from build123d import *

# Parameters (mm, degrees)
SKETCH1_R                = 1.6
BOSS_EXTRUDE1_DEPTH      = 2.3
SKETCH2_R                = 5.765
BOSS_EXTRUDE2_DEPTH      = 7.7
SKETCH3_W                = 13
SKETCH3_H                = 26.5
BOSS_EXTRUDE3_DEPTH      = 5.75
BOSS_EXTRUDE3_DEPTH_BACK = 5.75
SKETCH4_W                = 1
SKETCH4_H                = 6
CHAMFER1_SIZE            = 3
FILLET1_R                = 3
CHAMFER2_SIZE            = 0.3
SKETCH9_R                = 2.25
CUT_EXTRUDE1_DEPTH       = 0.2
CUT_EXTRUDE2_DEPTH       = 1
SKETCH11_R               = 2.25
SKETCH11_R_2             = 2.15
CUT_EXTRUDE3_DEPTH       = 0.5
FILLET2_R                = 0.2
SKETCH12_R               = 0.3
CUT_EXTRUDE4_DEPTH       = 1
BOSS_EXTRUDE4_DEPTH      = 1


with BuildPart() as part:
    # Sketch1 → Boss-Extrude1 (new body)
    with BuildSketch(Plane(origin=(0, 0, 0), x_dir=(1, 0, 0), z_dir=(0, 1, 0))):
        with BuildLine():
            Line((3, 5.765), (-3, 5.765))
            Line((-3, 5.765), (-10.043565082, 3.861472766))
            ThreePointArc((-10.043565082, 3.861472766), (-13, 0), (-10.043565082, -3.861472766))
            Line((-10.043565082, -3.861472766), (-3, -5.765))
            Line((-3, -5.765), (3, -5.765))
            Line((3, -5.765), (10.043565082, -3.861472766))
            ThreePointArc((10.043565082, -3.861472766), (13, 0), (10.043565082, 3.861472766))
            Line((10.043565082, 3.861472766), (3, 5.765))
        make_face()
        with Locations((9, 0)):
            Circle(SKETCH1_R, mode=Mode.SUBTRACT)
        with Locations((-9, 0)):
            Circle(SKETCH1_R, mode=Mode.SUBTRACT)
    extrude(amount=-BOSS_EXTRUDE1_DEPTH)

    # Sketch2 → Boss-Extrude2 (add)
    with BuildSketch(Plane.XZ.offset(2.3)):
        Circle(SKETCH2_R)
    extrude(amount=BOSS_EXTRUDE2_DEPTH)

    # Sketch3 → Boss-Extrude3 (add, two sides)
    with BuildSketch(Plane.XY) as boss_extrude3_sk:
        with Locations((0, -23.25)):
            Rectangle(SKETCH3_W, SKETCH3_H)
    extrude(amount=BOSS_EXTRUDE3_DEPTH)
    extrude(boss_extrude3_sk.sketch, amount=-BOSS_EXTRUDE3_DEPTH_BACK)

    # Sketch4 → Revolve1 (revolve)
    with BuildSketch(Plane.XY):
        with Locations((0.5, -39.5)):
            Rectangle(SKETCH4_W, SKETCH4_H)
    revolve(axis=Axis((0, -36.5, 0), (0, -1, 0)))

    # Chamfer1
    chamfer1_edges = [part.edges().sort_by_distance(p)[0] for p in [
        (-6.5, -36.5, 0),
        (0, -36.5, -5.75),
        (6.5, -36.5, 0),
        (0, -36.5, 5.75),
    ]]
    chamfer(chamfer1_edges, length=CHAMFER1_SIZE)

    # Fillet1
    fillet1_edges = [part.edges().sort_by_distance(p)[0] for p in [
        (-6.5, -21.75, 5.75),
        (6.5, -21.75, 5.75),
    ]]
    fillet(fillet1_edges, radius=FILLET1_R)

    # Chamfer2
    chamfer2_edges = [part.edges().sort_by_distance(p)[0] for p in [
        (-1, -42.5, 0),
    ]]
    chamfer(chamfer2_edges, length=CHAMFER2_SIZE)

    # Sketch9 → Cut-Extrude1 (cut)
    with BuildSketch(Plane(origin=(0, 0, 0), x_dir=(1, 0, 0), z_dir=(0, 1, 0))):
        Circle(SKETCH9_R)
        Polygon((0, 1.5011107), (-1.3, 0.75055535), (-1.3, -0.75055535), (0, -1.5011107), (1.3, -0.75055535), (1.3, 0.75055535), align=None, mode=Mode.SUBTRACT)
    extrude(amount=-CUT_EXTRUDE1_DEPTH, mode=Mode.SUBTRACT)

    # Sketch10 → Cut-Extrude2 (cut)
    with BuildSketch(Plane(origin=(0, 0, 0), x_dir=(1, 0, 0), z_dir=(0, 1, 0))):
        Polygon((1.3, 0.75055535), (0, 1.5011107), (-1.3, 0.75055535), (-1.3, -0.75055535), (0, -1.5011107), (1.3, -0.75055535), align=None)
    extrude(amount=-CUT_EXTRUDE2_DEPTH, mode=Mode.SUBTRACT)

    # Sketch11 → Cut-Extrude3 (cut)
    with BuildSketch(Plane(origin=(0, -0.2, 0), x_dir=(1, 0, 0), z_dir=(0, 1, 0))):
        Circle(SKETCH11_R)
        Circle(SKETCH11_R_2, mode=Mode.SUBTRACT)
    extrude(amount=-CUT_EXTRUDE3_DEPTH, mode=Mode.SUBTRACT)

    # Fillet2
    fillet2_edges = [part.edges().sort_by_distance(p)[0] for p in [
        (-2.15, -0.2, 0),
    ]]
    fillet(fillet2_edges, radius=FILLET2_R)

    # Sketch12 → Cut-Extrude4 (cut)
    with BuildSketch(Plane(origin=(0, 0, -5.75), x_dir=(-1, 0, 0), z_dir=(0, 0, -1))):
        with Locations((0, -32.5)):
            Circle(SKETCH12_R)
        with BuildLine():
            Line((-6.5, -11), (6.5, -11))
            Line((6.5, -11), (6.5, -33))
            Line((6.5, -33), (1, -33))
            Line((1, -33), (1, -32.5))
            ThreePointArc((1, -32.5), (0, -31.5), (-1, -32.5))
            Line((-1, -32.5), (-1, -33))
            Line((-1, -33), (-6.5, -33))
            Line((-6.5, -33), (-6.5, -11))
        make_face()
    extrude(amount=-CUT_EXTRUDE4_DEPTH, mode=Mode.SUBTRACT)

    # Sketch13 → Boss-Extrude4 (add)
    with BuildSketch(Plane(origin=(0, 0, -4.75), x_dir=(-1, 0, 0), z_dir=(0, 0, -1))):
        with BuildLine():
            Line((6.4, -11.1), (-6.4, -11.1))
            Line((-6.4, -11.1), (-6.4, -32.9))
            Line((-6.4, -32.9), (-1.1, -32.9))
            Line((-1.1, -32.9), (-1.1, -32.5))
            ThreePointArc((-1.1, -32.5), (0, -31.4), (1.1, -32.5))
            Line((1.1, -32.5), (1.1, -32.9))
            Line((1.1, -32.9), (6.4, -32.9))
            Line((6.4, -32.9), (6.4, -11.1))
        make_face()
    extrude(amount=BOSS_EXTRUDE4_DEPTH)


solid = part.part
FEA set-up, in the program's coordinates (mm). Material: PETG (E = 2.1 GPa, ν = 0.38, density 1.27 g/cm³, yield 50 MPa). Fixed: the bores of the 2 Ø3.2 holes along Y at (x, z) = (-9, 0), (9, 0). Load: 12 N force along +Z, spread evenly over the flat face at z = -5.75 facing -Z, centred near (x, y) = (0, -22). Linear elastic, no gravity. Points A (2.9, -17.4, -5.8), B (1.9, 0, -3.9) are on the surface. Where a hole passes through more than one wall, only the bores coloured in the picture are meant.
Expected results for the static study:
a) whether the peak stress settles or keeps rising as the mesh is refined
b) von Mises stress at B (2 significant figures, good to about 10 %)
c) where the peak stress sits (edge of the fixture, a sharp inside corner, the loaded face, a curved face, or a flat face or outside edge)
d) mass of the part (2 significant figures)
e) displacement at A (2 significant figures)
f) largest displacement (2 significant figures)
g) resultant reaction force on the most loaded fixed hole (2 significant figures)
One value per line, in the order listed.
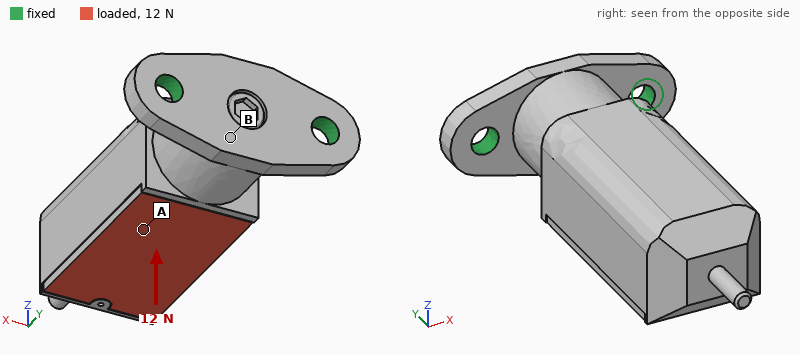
keeps rising
2.7 MPa
edge of the fixture
6.4 g
0.23 mm
0.56 mm
6.0 N
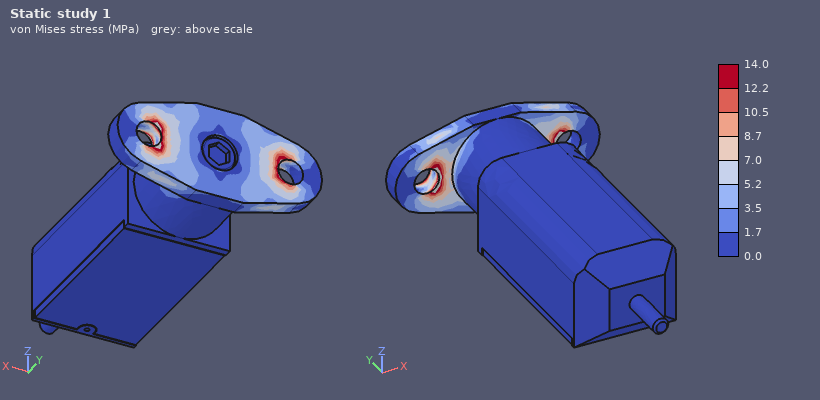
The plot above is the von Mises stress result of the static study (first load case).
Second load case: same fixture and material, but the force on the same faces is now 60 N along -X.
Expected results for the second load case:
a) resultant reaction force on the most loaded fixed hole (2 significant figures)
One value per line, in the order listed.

99 N
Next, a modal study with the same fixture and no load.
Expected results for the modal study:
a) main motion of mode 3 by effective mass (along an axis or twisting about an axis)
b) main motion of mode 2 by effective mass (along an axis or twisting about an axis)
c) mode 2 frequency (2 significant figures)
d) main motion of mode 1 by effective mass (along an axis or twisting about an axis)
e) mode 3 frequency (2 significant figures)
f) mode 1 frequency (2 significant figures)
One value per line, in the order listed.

along Y
along X
1000 Hz
along Z
3600 Hz
430 Hz
